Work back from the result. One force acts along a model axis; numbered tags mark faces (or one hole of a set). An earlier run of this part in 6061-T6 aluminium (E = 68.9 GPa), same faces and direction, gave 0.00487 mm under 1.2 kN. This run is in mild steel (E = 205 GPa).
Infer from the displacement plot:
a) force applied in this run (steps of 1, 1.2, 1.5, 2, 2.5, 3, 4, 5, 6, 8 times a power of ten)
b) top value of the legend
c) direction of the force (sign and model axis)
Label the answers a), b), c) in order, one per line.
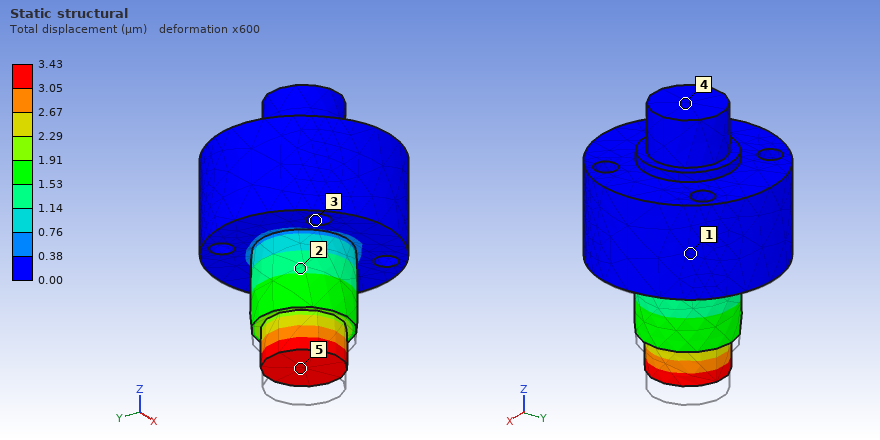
a) 2.5 kN
b) 3.43 µm
c) +Z
